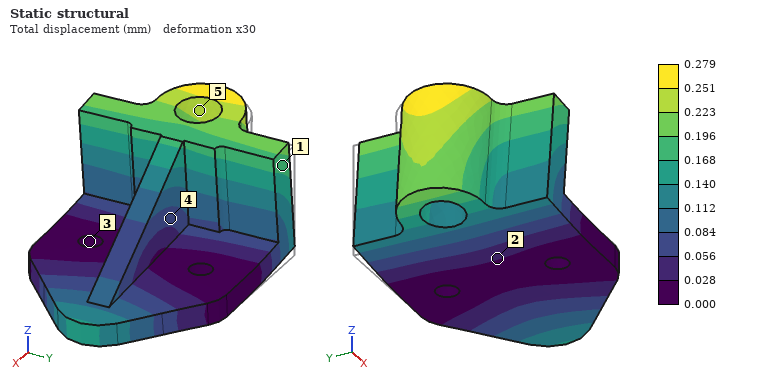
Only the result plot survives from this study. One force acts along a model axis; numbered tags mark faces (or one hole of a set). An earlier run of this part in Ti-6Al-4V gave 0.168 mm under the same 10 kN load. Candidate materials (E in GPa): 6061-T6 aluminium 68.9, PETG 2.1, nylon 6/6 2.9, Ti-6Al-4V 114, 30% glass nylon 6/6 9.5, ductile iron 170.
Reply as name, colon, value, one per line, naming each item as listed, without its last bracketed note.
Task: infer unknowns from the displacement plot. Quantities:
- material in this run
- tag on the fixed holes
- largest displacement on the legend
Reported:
material in this run: 6061-T6 aluminium
tag on the fixed holes: 3
largest displacement on the legend: 0.279 mm
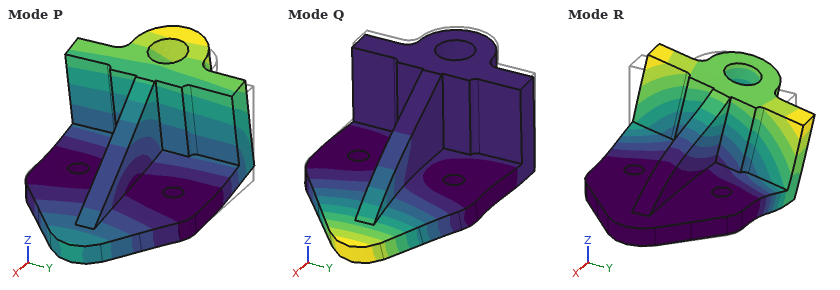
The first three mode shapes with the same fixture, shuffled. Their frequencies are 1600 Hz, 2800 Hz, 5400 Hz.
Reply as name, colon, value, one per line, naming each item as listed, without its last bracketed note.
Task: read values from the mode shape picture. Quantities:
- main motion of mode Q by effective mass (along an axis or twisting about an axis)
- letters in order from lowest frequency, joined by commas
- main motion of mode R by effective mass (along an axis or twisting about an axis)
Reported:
main motion of mode Q by effective mass: along Z
letters in order from lowest frequency, joined by commas: P, R, Q
main motion of mode R by effective mass: along Y
